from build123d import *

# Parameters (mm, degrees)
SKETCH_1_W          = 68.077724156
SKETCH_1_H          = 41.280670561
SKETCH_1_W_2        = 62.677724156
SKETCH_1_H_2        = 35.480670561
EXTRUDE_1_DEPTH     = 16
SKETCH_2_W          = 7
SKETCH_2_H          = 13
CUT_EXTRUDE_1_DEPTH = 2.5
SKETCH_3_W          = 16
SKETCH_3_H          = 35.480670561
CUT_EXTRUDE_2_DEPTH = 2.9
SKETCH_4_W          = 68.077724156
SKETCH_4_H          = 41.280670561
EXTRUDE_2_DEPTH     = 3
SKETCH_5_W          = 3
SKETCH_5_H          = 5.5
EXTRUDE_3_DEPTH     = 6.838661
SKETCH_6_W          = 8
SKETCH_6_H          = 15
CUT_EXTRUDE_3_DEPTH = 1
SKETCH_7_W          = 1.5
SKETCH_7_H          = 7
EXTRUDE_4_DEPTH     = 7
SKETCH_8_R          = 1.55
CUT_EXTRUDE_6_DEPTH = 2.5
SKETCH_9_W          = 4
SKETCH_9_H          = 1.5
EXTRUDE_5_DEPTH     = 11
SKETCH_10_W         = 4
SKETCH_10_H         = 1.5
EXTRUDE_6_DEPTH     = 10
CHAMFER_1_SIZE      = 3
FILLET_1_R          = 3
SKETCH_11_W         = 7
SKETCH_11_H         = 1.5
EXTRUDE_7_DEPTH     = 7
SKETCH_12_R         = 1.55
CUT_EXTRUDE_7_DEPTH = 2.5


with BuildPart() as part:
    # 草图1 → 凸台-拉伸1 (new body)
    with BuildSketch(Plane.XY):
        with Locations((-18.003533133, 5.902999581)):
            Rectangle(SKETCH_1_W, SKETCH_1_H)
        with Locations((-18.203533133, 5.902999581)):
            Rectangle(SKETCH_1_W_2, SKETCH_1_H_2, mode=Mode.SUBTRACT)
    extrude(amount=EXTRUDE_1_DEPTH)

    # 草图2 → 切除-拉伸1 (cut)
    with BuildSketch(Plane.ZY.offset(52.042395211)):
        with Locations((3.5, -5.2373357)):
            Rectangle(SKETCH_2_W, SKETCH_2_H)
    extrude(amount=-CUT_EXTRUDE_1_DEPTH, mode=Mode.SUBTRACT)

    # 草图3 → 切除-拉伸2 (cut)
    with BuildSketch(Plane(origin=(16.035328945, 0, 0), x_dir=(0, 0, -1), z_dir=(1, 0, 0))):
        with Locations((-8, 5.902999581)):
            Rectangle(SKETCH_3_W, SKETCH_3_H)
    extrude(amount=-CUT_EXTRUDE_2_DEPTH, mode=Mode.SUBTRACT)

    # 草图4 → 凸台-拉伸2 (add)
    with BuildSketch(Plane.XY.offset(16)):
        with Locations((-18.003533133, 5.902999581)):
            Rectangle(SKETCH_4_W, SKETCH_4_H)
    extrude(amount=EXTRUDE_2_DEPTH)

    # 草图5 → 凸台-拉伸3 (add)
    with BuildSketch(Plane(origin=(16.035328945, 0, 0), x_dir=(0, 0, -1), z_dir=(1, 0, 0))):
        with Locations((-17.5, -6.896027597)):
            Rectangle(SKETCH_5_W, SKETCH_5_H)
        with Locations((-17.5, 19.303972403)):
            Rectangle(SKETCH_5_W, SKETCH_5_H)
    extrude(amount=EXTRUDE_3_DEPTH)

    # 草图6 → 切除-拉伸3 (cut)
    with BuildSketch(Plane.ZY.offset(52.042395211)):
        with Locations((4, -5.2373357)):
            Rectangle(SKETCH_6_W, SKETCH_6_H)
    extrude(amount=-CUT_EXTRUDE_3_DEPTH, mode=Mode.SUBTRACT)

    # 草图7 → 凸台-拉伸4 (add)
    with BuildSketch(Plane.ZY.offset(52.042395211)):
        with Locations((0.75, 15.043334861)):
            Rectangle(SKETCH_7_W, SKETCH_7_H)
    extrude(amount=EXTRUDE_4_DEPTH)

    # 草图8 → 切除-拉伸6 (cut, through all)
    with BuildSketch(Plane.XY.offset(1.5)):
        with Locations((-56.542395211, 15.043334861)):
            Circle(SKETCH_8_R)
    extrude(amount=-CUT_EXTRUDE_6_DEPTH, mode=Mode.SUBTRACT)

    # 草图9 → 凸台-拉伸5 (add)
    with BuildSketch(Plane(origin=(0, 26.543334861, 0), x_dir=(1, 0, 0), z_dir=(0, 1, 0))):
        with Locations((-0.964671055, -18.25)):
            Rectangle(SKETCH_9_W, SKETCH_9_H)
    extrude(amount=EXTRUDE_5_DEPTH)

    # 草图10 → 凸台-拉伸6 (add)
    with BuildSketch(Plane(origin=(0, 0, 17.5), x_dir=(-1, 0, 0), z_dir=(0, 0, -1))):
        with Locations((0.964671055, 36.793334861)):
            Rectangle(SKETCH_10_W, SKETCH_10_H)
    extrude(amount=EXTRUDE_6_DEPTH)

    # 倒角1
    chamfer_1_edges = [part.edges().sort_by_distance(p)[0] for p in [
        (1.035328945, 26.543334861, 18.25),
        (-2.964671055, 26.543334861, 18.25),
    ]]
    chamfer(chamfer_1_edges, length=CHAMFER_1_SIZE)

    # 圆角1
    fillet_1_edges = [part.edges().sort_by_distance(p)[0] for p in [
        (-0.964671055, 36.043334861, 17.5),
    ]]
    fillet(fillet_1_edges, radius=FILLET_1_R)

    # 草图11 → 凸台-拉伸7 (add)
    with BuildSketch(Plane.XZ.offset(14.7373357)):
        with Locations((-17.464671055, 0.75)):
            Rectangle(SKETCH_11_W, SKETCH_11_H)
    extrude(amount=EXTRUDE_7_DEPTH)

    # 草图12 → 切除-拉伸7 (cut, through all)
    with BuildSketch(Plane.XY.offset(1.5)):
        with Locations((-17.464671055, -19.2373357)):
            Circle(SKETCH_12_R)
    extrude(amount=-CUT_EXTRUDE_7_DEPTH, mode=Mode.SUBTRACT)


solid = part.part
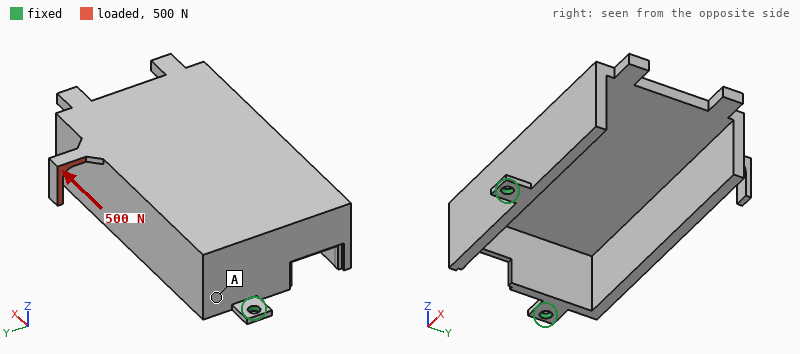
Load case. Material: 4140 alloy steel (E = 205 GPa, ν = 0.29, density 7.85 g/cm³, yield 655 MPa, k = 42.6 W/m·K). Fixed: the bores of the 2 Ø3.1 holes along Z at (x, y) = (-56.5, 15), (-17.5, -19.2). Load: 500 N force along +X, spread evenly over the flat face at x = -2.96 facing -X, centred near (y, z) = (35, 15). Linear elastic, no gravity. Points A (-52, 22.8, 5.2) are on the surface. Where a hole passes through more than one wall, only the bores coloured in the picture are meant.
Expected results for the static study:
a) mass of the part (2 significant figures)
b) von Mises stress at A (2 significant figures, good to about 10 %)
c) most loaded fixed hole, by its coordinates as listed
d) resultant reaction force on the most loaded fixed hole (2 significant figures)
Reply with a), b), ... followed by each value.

a) 130 g
b) 82 MPa
c) (-56.5, 15)
d) 570 N
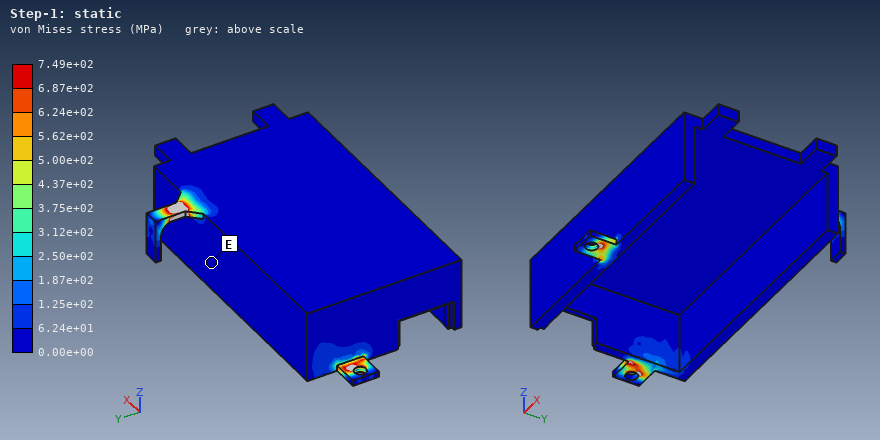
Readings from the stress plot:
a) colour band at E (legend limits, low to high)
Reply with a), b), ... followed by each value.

a) 0.00e+00 to 6.24e+01 MPa
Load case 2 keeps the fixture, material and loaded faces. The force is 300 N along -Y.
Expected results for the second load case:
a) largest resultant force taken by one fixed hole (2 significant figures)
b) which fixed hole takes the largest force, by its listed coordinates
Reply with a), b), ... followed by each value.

a) 300 N
b) (-17.5, -19.2)
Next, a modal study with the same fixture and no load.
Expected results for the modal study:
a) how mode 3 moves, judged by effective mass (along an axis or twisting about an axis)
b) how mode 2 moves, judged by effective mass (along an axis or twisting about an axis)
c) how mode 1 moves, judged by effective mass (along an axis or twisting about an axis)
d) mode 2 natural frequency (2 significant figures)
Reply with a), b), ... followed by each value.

a) along X
b) along Y
c) along Z
d) 1300 Hz
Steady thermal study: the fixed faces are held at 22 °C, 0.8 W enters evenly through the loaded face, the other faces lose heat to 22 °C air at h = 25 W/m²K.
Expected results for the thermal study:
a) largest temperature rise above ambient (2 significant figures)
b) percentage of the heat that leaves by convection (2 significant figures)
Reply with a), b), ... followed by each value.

a) 32 K
b) 81 %
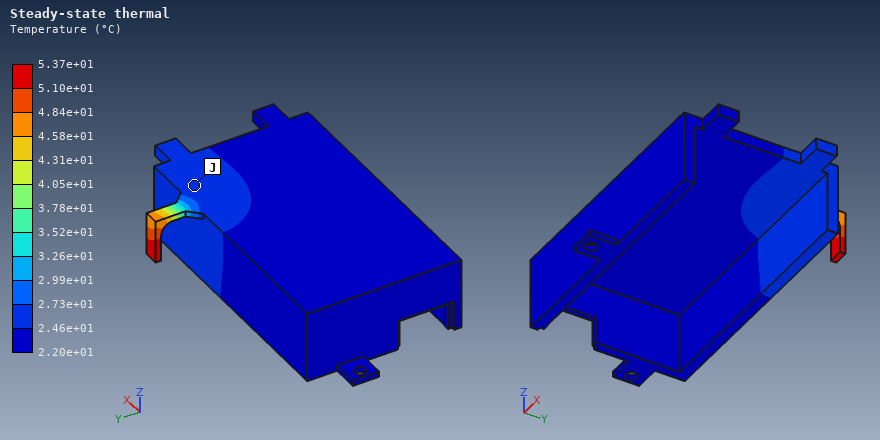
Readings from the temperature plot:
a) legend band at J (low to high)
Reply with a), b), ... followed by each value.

a) 2.46e+01 to 2.73e+01 °C
